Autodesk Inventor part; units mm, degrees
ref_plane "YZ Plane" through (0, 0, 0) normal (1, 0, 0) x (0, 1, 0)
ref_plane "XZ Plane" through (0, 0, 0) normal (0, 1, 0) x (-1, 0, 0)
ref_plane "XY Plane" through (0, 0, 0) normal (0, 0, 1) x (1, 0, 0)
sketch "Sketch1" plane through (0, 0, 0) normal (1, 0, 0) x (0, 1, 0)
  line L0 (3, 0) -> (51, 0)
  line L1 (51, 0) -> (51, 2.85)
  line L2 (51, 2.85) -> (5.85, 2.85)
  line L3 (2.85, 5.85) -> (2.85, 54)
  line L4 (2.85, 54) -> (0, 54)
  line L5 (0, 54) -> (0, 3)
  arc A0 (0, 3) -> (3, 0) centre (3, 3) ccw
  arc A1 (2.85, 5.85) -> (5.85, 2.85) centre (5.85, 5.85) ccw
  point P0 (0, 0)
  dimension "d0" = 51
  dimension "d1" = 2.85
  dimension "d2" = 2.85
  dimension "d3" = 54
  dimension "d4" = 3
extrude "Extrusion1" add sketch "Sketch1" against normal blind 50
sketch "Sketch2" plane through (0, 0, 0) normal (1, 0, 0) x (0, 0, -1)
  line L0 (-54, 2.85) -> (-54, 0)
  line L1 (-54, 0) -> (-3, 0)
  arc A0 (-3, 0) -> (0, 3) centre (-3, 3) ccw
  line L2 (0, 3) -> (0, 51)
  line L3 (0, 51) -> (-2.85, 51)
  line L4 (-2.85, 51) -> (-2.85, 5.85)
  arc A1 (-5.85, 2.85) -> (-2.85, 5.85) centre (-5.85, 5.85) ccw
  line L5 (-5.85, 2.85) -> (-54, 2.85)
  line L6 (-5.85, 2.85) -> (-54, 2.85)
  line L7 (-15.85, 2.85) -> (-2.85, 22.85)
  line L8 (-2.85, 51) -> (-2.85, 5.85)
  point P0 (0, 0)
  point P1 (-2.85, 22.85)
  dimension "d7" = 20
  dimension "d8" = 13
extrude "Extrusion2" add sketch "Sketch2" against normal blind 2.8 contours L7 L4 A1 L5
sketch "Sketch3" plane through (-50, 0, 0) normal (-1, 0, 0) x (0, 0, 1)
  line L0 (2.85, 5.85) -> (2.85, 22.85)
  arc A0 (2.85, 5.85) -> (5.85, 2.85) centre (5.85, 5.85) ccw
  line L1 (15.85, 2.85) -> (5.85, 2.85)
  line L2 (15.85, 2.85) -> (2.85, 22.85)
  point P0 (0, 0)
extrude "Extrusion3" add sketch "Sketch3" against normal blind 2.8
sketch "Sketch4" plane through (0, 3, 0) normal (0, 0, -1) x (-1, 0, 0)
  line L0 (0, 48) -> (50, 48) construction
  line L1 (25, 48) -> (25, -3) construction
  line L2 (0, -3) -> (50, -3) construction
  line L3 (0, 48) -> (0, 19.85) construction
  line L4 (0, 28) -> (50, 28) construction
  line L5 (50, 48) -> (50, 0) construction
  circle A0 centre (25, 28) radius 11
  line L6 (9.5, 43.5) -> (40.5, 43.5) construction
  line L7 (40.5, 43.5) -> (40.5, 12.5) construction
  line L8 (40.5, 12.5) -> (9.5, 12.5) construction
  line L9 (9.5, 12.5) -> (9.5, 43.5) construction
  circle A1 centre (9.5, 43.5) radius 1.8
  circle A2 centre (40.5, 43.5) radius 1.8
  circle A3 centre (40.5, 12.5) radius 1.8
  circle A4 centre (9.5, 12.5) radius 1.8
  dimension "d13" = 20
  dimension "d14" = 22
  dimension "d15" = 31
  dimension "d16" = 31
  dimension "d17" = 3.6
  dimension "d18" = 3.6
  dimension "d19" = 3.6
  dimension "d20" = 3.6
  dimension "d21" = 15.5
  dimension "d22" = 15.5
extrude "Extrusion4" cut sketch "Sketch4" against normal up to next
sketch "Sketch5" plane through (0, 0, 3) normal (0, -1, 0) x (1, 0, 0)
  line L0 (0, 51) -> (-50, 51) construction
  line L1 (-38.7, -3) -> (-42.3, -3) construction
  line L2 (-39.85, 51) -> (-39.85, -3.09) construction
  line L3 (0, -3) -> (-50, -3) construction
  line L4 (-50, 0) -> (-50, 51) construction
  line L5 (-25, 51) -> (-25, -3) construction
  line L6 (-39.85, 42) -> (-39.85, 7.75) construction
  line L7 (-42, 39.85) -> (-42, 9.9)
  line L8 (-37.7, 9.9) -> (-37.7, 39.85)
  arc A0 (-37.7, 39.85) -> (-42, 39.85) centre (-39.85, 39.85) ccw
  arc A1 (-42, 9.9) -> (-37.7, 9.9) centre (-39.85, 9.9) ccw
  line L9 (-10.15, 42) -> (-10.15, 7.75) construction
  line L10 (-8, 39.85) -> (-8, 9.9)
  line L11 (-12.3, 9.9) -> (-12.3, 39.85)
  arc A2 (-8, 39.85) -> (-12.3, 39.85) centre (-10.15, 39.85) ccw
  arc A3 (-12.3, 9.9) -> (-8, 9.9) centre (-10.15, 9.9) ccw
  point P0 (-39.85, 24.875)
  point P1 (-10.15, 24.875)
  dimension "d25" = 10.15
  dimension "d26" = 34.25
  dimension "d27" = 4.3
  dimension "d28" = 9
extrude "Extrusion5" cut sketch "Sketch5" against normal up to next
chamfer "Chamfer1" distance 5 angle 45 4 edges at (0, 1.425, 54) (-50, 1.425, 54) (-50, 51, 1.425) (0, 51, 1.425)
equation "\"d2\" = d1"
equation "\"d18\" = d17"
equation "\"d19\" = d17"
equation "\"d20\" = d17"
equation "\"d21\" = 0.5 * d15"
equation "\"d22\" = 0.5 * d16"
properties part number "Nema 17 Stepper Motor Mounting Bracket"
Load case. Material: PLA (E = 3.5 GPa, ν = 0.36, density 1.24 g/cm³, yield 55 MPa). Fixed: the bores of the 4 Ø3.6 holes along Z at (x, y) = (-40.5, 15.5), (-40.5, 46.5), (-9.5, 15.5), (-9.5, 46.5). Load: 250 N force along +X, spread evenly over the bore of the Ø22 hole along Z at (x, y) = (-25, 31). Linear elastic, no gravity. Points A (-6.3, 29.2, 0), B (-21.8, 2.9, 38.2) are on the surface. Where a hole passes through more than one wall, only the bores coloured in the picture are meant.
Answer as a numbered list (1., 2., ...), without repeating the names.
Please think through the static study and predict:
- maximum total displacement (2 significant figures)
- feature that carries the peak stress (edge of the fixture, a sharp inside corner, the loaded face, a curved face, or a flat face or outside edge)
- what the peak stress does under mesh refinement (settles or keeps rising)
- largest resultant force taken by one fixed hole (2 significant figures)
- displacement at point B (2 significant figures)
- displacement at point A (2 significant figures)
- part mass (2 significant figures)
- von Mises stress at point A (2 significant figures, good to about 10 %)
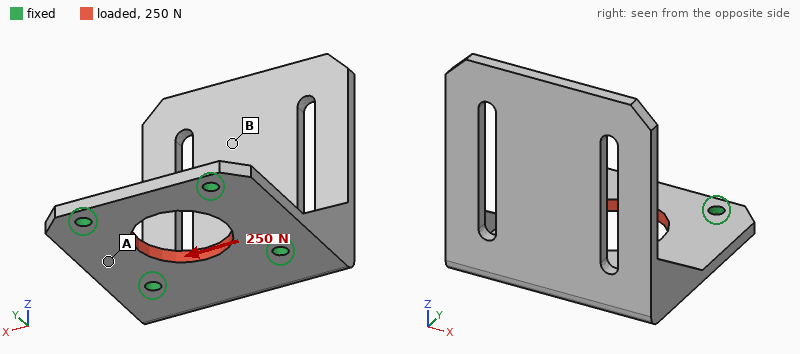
1. 12 µm
2. edge of the fixture
3. keeps rising
4. 66 N
5. 2.3 µm
6. 9.9 µm
7. 16 g
8. 0.89 MPa
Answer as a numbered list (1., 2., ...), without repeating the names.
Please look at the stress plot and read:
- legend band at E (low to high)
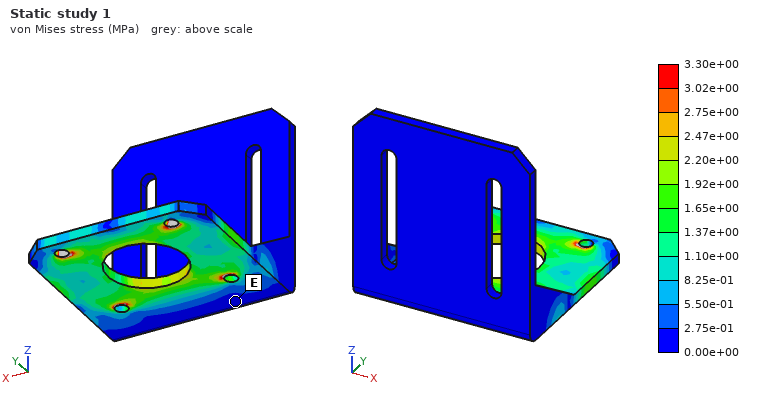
1. 0.00e+00 to 2.75e-01 MPa
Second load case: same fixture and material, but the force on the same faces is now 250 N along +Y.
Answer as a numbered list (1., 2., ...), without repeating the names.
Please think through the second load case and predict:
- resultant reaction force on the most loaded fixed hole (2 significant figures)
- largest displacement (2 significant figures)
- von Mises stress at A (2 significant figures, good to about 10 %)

1. 66 N
2. 17 µm
3. 0.70 MPa
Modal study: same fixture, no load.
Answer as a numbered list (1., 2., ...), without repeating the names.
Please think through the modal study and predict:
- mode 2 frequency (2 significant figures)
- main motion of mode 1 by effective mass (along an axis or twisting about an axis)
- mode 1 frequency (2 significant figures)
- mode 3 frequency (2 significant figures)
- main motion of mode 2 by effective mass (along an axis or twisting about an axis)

1. 650 Hz
2. along Y
3. 290 Hz
4. 990 Hz
5. along X
